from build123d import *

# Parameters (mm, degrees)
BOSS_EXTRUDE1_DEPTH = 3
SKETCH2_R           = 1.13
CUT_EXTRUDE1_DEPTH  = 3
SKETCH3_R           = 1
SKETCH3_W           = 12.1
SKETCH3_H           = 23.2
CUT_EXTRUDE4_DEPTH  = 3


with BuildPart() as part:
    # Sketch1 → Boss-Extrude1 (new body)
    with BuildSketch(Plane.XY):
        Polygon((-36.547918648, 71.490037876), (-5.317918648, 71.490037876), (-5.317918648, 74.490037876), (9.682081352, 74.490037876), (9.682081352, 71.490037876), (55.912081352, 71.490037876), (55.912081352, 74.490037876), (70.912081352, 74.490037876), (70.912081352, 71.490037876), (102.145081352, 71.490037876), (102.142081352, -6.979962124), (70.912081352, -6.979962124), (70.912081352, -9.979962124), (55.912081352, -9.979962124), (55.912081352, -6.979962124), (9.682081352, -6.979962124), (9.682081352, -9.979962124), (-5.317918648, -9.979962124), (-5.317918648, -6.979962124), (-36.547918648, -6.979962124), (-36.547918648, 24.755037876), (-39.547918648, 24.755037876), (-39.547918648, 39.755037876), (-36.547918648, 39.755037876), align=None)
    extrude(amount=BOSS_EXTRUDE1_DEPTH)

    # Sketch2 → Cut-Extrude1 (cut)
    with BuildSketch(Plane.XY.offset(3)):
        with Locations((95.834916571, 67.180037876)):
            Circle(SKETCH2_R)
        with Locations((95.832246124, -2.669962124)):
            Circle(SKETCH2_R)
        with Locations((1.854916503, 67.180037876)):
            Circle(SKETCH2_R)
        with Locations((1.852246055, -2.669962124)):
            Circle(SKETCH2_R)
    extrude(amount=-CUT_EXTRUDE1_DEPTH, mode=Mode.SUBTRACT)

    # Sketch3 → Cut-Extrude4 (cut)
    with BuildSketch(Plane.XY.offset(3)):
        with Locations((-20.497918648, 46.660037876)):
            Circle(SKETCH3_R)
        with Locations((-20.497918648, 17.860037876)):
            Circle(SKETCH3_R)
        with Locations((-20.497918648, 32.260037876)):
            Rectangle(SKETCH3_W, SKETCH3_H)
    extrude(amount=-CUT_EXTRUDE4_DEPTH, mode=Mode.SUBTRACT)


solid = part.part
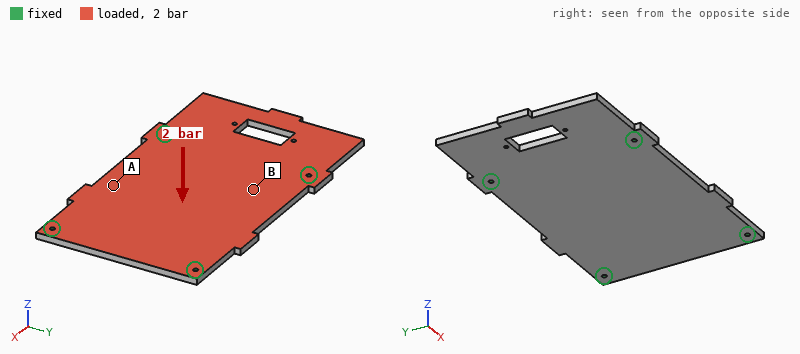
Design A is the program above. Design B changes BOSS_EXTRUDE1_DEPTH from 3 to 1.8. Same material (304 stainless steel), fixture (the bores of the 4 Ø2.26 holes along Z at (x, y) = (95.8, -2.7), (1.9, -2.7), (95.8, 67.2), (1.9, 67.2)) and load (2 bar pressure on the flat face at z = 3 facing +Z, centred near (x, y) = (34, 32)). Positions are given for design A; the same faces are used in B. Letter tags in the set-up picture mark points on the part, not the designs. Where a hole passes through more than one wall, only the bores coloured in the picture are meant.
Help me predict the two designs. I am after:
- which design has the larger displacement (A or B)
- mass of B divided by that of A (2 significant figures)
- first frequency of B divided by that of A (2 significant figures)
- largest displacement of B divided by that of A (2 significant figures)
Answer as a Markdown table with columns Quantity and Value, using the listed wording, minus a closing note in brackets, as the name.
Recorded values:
| Quantity | Value |
|---|---|
| which design has the larger displacement | B |
| mass of B divided by that of A | 0.60 |
| first frequency of B divided by that of A | 0.62 |
| largest displacement of B divided by that of A | 4.5 |
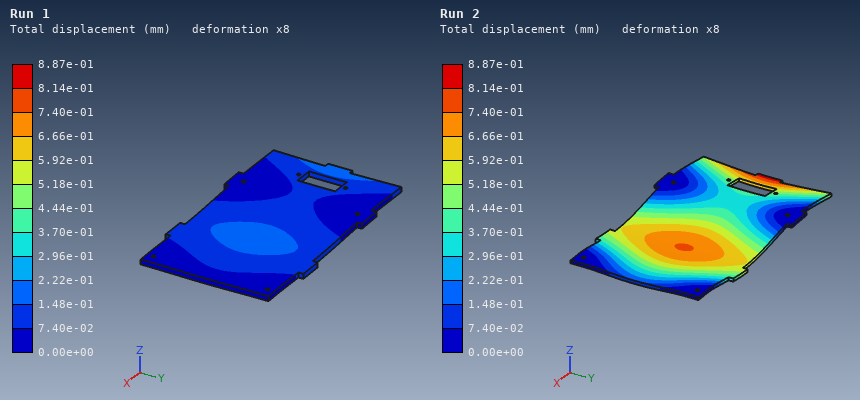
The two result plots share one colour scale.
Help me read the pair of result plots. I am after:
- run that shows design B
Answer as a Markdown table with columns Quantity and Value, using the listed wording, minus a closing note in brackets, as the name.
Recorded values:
| Quantity | Value |
|---|---|
| run that shows design B | Run 2 |
